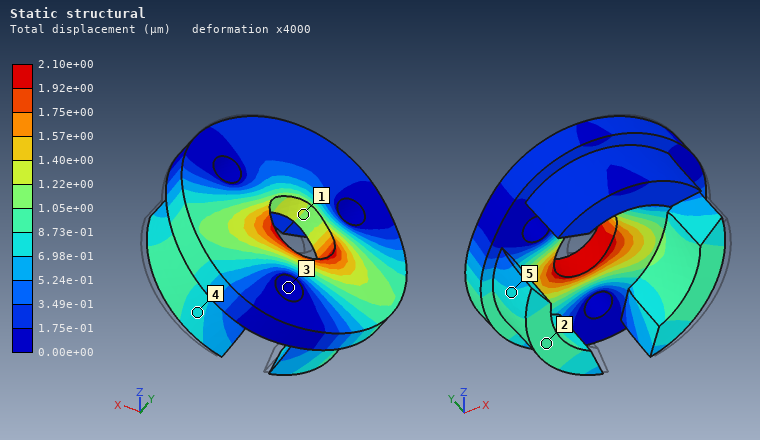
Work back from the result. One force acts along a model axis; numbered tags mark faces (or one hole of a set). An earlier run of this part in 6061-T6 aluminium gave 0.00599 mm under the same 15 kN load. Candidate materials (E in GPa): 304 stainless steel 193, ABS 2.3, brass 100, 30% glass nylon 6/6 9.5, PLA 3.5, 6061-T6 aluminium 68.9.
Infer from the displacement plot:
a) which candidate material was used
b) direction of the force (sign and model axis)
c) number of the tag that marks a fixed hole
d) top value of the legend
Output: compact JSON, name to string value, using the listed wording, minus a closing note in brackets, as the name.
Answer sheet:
{"which candidate material was used": "304 stainless steel", "direction of the force": "-X", "number of the tag that marks a fixed hole": "3", "top value of the legend": "2.10e+00 µm"}
